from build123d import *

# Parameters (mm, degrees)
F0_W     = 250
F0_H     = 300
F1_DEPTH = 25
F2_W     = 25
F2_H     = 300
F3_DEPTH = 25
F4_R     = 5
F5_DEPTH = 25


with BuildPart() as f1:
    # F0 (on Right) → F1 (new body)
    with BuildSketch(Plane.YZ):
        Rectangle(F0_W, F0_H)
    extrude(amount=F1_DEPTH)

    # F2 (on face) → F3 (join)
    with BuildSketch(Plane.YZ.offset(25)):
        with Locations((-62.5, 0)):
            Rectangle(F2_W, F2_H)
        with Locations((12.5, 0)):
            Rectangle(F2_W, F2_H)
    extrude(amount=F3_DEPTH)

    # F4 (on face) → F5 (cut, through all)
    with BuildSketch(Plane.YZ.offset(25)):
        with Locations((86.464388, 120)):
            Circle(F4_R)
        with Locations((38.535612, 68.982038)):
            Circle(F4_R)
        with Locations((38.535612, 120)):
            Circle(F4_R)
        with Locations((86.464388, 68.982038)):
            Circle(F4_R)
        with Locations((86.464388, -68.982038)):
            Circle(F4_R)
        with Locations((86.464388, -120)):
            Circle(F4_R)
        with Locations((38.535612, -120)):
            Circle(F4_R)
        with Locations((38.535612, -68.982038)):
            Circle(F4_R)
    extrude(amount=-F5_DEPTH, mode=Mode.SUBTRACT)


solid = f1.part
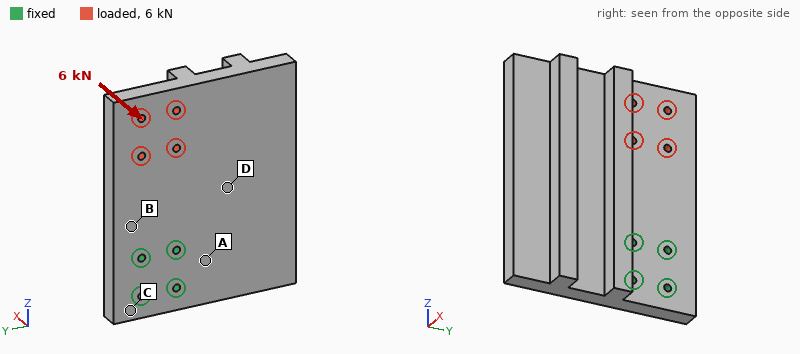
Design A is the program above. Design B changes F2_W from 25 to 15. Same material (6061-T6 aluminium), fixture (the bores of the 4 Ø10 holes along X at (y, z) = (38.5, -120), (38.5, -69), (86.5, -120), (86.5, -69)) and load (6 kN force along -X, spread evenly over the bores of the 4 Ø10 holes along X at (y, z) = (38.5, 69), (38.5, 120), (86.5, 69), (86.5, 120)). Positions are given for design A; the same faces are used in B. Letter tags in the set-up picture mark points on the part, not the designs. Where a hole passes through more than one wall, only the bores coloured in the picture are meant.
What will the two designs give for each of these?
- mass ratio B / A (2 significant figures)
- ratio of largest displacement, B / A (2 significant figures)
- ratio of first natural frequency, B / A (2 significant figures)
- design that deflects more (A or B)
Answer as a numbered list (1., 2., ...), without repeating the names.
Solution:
1. 0.93
2. 1.2
3. 0.97
4. B
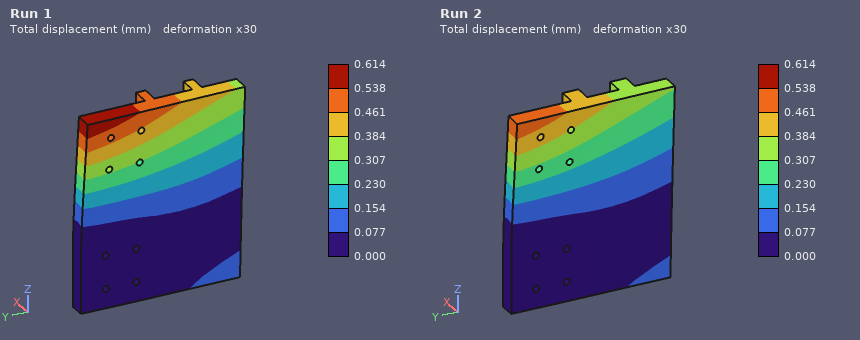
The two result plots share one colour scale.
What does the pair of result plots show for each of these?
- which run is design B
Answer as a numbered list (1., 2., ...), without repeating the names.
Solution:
1. Run 1
